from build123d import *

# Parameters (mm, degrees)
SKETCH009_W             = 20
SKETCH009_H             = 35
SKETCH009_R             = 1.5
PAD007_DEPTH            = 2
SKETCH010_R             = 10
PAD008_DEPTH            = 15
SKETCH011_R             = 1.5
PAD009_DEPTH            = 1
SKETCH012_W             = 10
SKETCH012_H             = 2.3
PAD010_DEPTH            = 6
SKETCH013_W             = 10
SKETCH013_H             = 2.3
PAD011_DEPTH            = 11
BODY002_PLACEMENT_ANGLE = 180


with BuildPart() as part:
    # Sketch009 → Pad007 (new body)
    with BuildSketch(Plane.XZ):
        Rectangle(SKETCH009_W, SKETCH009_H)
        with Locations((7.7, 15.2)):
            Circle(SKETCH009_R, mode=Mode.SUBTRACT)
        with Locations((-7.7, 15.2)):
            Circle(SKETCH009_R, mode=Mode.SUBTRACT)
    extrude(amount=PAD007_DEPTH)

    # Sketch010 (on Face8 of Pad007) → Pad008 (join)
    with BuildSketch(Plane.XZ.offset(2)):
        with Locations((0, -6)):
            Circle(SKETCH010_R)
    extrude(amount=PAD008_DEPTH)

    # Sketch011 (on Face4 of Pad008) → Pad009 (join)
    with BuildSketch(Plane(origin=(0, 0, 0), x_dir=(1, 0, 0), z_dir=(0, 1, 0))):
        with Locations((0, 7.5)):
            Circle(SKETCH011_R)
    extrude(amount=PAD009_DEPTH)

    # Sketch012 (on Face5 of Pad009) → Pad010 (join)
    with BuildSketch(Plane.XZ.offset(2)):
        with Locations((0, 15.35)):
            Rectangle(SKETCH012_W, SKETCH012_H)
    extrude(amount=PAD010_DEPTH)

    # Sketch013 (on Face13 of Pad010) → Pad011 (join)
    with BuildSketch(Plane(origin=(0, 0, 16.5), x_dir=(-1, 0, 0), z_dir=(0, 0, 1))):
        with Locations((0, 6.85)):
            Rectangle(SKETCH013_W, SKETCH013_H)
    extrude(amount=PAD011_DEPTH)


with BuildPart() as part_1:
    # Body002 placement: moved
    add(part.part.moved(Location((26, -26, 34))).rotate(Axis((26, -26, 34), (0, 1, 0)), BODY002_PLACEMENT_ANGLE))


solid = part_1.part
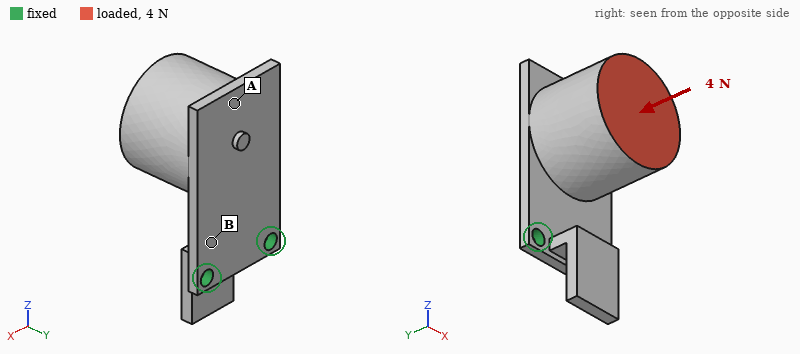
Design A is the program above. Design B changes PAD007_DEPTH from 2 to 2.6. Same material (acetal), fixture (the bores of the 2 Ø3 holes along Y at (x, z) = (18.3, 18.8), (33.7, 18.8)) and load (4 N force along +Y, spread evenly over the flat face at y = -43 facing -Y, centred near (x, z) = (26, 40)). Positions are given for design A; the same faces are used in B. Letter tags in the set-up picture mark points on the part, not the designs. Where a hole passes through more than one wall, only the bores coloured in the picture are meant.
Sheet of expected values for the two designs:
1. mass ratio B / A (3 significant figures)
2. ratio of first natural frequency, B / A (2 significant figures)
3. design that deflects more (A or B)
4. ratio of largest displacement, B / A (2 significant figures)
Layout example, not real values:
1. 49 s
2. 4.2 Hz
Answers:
1. 1.03
2. 1.4
3. A
4. 0.48
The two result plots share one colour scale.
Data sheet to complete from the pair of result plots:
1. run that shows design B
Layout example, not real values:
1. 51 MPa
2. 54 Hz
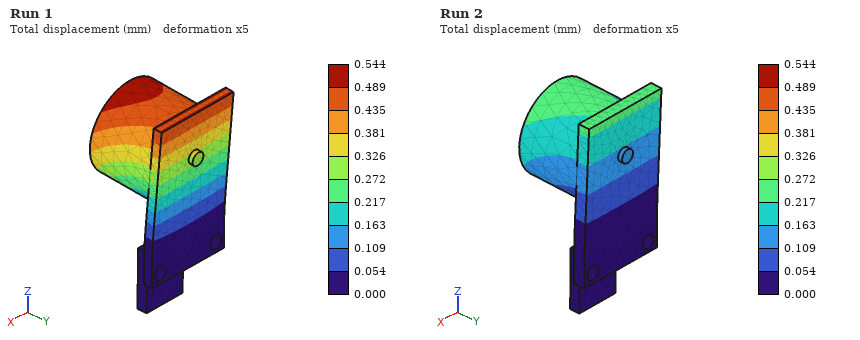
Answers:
1. Run 2
